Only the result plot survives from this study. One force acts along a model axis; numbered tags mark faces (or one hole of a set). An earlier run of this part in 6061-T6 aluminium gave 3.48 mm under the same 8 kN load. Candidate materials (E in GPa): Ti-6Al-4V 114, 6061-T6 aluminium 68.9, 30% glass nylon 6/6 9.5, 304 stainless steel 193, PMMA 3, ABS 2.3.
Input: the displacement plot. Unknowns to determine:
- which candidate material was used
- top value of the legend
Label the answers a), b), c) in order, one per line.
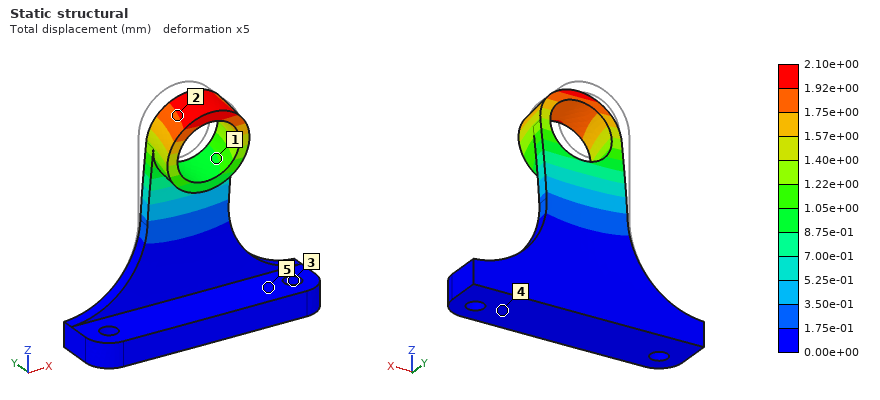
a) Ti-6Al-4V
b) 2.10e+00 mm
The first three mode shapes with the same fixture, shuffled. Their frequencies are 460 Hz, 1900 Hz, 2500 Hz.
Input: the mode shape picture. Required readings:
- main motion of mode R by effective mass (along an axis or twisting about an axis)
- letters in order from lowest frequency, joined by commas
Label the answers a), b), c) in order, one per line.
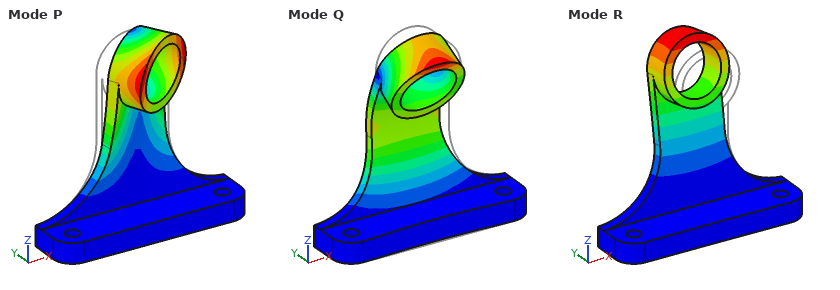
a) along Y
b) R, P, Q
